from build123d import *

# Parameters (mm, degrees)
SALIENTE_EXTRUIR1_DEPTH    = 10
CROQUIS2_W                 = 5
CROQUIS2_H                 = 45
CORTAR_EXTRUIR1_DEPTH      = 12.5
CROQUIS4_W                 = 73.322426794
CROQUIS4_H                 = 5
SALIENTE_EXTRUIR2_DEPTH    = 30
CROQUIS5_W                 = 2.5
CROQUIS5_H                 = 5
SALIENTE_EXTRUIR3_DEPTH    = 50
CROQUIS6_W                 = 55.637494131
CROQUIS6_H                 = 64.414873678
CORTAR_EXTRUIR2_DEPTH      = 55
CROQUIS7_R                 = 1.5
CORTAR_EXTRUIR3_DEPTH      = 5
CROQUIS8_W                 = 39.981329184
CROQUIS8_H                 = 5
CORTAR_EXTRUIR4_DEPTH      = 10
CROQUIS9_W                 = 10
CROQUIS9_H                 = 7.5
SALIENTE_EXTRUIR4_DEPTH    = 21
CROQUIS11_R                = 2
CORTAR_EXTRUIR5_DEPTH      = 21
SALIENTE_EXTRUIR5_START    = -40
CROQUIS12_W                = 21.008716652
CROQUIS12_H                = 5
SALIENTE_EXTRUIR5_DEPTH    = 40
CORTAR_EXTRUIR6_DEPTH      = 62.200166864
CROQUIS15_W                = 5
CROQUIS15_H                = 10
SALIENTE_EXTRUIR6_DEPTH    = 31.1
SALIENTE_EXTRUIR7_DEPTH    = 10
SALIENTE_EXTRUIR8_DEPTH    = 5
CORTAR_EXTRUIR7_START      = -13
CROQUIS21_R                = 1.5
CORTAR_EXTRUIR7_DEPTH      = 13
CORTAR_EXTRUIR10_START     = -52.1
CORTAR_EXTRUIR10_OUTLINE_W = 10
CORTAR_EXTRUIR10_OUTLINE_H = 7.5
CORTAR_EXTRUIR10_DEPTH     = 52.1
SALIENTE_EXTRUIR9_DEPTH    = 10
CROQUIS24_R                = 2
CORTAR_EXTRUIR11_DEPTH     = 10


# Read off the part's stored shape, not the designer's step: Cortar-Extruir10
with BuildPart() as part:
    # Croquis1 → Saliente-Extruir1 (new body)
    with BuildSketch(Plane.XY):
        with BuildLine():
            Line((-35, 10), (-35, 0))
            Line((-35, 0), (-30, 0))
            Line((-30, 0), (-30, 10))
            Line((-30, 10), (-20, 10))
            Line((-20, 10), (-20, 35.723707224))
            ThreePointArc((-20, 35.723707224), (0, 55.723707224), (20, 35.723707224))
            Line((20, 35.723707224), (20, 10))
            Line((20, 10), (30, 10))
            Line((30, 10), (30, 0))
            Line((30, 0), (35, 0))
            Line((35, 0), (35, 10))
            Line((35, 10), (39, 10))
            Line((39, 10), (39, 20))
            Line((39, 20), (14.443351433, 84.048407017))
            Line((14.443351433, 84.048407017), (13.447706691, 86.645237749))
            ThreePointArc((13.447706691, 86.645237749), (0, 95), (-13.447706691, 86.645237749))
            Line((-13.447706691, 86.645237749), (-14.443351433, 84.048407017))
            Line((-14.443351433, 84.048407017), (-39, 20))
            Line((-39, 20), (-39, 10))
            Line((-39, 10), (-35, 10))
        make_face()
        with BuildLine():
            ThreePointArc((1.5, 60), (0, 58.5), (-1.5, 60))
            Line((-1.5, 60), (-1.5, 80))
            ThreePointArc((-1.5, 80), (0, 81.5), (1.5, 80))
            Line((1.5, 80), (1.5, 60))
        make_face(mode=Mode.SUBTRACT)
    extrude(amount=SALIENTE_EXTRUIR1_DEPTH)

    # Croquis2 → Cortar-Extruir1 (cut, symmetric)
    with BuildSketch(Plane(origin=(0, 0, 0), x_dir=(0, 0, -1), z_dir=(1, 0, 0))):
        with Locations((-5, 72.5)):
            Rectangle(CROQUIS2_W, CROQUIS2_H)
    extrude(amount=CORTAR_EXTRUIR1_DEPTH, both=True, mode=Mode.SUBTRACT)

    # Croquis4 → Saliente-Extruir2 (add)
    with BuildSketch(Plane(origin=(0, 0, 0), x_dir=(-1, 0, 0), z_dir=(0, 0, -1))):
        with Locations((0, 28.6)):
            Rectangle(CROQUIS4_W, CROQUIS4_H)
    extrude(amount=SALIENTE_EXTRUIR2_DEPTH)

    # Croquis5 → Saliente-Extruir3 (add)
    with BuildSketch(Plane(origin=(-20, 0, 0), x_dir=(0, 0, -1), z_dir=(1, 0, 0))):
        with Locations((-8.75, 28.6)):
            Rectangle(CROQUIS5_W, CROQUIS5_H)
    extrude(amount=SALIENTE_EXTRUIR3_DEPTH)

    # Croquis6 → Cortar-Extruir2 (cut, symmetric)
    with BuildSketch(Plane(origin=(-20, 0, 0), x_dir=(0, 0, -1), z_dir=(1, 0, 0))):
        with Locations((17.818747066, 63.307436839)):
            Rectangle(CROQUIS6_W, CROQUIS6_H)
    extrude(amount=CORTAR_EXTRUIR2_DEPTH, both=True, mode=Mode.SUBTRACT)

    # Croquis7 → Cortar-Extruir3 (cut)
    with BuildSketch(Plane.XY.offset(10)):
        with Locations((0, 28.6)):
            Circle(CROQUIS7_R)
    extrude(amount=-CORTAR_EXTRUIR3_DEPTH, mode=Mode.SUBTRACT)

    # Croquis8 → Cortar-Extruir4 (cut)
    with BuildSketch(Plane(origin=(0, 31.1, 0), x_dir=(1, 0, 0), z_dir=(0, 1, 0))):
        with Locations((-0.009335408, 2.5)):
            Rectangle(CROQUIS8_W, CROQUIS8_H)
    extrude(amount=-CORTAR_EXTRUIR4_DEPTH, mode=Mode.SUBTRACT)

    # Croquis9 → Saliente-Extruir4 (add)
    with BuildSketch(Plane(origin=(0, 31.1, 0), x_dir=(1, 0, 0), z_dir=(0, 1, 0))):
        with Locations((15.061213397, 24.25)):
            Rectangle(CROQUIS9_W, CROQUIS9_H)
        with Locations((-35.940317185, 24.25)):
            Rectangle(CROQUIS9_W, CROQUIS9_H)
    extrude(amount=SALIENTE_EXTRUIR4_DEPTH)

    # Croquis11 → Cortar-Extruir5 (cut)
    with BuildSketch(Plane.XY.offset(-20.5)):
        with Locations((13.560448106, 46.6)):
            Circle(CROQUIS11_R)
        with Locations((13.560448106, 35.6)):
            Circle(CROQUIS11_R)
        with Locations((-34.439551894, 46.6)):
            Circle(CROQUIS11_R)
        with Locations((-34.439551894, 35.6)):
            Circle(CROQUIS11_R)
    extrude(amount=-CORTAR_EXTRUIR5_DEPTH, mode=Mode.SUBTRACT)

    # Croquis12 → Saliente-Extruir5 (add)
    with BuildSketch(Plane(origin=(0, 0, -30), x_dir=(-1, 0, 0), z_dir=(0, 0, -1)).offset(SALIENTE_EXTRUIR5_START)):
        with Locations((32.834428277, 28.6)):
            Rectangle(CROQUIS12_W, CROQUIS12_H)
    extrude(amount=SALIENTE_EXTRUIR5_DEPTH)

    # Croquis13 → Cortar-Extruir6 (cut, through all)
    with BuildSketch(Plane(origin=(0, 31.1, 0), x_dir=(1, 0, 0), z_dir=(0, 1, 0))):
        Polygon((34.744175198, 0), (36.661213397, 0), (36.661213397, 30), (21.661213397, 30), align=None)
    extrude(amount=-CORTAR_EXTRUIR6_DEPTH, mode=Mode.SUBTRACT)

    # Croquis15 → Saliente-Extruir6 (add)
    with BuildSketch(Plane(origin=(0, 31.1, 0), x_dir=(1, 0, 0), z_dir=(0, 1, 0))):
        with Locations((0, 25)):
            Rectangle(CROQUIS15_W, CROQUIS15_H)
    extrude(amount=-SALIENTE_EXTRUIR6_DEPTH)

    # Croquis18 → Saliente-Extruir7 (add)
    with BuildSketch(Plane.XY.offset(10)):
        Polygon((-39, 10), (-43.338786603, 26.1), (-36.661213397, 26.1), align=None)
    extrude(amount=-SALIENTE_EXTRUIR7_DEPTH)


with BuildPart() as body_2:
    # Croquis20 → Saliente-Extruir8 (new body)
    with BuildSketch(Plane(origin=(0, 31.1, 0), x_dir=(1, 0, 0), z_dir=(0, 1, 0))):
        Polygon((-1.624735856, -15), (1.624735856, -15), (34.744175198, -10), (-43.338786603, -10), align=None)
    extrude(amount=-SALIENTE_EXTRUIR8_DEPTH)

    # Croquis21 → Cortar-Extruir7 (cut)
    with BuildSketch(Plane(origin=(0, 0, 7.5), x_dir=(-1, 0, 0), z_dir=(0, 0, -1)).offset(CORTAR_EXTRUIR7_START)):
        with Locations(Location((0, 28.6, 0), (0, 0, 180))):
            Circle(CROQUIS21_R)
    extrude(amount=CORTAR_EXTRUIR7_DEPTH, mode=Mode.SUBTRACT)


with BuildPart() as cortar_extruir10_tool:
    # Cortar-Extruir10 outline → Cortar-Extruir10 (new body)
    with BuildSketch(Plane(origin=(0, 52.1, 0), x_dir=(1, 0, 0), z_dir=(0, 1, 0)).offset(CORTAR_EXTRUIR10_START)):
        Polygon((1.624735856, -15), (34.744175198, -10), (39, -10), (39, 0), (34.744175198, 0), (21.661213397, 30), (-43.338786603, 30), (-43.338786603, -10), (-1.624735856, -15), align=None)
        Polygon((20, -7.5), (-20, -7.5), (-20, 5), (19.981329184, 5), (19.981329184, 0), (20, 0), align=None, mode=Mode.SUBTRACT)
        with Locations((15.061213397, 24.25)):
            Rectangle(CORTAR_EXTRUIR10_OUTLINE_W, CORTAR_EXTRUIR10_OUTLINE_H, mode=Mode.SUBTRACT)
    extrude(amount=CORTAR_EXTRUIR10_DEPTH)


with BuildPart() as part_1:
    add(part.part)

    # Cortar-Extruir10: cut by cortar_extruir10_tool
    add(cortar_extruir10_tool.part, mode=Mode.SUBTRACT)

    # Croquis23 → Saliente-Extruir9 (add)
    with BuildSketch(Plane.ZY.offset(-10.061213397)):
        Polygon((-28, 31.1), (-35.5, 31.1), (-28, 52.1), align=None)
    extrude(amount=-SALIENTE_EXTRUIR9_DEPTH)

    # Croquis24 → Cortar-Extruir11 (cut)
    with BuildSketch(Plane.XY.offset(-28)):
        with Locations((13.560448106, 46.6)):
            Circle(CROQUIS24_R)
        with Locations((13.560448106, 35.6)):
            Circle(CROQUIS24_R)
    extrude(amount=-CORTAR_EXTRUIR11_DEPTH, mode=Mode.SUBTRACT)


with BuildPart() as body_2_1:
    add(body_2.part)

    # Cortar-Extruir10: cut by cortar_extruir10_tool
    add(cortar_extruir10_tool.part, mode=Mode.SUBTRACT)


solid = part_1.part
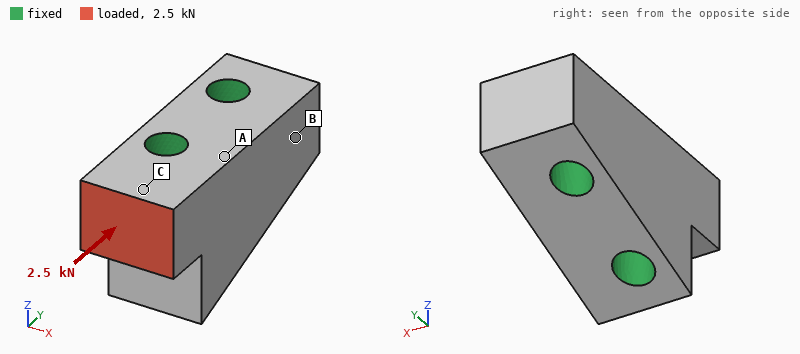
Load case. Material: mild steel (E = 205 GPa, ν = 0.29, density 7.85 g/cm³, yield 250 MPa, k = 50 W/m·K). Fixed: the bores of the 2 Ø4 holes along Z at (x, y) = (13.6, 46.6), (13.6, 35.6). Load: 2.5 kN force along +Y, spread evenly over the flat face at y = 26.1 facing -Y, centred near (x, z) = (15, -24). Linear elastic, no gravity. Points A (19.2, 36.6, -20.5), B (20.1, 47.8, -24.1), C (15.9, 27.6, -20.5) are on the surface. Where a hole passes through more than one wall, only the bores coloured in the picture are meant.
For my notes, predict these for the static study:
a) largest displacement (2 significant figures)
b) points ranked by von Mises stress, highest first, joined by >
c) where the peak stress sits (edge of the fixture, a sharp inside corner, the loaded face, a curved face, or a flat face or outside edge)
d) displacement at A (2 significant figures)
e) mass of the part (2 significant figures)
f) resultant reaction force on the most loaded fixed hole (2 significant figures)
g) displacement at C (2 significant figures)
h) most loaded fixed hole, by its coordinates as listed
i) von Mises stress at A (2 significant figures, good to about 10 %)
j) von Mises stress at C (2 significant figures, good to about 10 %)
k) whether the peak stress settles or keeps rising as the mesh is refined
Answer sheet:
2.4 µm
C > A > B
edge of the fixture
0.59 µm
19 g
2.3 kN
1.7 µm
(13.6, 35.6)
23 MPa
35 MPa
keeps rising
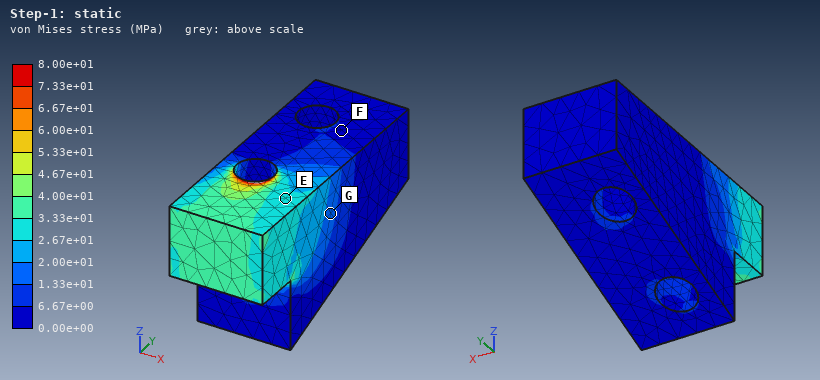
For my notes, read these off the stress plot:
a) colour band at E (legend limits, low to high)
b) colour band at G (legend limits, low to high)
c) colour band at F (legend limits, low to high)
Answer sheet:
2.67e+01 to 3.33e+01 MPa
1.33e+01 to 2.00e+01 MPa
0.00e+00 to 6.67e+00 MPa
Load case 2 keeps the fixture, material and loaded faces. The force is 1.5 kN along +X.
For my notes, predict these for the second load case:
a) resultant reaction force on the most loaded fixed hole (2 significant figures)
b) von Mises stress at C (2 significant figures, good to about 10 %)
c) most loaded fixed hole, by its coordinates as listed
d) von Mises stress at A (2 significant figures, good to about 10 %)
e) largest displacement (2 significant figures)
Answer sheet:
2.0 kN
52 MPa
(13.6, 35.6)
43 MPa
7.5 µm
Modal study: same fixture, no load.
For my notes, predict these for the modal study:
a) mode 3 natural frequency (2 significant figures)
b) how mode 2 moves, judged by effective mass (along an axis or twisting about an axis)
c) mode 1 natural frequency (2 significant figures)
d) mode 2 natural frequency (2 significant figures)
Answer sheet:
93 kHz
along Z
57 kHz
68 kHz
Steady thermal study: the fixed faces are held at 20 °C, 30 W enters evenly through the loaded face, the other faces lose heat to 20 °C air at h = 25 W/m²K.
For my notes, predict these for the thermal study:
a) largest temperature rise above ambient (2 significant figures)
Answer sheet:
66 K
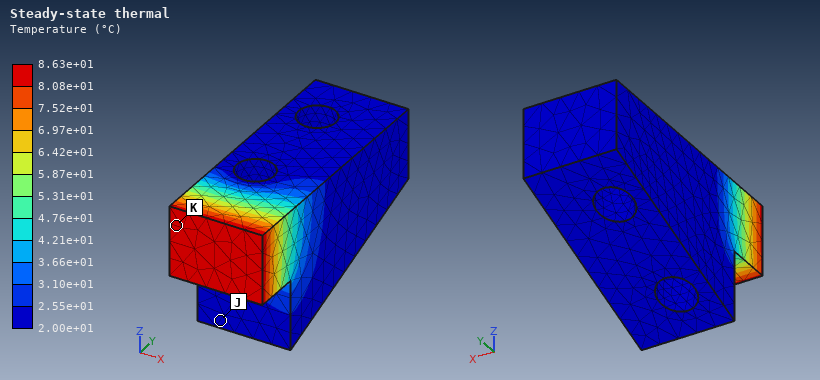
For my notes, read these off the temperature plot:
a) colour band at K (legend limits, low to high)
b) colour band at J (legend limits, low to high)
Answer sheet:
8.08e+01 to 8.63e+01 °C
2.00e+01 to 2.55e+01 °C
